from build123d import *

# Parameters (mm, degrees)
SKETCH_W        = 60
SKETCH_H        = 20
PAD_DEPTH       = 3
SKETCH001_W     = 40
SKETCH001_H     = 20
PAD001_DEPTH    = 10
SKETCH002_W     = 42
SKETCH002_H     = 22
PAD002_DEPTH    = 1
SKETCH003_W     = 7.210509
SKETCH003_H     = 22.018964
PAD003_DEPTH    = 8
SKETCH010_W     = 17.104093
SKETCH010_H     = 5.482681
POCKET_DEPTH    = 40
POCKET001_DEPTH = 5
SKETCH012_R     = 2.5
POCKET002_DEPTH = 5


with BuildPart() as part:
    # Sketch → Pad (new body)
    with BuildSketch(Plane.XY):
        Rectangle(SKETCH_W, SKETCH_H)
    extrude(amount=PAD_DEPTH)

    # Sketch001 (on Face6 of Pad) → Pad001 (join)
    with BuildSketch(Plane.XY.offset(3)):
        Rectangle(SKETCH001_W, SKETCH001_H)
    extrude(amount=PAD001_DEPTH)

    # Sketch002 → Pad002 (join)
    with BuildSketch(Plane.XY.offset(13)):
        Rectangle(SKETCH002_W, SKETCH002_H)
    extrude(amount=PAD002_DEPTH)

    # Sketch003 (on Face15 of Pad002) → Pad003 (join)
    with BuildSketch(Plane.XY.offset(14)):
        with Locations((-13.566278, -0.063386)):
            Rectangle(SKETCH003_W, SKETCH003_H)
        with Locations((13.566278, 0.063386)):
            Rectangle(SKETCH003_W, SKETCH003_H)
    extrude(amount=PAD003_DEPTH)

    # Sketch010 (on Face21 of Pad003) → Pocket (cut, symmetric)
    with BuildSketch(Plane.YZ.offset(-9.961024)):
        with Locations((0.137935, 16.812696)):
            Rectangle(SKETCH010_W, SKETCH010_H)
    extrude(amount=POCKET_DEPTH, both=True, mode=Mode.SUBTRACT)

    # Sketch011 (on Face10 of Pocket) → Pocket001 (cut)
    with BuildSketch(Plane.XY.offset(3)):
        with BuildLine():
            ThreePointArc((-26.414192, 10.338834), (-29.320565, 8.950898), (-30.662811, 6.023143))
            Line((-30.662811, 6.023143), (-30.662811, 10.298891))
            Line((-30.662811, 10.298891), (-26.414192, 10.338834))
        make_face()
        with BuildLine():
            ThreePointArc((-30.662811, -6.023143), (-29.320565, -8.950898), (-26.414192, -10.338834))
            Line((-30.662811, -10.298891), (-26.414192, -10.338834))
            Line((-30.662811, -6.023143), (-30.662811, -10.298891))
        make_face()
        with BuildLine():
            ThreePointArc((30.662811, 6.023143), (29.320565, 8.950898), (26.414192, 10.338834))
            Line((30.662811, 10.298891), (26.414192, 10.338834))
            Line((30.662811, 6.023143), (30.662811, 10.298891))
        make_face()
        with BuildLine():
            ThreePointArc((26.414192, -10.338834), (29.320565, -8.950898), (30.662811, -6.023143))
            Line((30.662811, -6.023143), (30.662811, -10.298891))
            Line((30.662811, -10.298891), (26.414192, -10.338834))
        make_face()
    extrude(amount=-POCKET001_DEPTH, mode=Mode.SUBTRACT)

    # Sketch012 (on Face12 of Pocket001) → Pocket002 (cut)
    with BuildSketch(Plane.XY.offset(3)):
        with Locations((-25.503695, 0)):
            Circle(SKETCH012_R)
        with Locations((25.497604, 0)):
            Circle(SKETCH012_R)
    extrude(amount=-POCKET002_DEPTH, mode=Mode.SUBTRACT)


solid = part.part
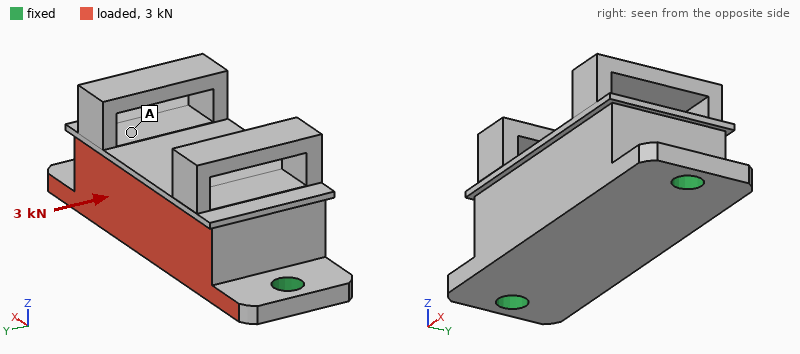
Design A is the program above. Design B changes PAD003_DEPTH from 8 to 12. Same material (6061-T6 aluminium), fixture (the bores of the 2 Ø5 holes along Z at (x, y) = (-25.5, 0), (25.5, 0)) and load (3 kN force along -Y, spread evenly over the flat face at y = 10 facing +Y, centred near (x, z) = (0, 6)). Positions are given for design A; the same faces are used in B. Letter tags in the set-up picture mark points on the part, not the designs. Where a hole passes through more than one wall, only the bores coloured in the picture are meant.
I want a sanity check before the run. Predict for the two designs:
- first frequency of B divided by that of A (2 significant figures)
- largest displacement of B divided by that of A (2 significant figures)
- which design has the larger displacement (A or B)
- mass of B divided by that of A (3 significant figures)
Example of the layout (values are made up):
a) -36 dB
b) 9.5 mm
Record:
a) 0.81
b) 1.1
c) B
d) 1.09
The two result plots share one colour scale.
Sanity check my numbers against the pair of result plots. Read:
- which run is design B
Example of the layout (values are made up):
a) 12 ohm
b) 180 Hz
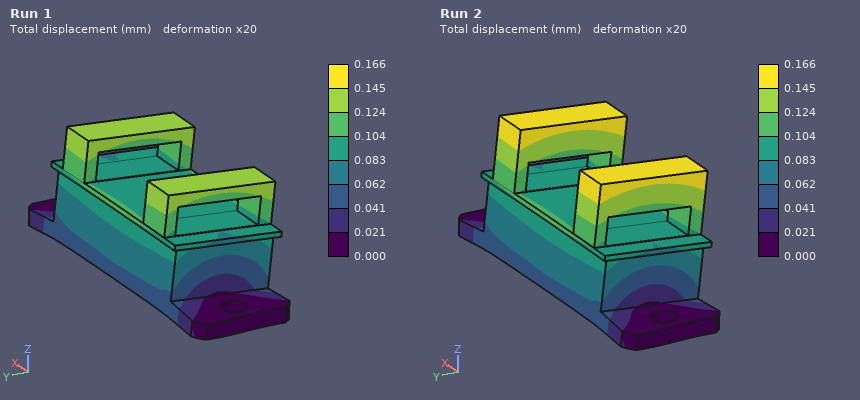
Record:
a) Run 2
